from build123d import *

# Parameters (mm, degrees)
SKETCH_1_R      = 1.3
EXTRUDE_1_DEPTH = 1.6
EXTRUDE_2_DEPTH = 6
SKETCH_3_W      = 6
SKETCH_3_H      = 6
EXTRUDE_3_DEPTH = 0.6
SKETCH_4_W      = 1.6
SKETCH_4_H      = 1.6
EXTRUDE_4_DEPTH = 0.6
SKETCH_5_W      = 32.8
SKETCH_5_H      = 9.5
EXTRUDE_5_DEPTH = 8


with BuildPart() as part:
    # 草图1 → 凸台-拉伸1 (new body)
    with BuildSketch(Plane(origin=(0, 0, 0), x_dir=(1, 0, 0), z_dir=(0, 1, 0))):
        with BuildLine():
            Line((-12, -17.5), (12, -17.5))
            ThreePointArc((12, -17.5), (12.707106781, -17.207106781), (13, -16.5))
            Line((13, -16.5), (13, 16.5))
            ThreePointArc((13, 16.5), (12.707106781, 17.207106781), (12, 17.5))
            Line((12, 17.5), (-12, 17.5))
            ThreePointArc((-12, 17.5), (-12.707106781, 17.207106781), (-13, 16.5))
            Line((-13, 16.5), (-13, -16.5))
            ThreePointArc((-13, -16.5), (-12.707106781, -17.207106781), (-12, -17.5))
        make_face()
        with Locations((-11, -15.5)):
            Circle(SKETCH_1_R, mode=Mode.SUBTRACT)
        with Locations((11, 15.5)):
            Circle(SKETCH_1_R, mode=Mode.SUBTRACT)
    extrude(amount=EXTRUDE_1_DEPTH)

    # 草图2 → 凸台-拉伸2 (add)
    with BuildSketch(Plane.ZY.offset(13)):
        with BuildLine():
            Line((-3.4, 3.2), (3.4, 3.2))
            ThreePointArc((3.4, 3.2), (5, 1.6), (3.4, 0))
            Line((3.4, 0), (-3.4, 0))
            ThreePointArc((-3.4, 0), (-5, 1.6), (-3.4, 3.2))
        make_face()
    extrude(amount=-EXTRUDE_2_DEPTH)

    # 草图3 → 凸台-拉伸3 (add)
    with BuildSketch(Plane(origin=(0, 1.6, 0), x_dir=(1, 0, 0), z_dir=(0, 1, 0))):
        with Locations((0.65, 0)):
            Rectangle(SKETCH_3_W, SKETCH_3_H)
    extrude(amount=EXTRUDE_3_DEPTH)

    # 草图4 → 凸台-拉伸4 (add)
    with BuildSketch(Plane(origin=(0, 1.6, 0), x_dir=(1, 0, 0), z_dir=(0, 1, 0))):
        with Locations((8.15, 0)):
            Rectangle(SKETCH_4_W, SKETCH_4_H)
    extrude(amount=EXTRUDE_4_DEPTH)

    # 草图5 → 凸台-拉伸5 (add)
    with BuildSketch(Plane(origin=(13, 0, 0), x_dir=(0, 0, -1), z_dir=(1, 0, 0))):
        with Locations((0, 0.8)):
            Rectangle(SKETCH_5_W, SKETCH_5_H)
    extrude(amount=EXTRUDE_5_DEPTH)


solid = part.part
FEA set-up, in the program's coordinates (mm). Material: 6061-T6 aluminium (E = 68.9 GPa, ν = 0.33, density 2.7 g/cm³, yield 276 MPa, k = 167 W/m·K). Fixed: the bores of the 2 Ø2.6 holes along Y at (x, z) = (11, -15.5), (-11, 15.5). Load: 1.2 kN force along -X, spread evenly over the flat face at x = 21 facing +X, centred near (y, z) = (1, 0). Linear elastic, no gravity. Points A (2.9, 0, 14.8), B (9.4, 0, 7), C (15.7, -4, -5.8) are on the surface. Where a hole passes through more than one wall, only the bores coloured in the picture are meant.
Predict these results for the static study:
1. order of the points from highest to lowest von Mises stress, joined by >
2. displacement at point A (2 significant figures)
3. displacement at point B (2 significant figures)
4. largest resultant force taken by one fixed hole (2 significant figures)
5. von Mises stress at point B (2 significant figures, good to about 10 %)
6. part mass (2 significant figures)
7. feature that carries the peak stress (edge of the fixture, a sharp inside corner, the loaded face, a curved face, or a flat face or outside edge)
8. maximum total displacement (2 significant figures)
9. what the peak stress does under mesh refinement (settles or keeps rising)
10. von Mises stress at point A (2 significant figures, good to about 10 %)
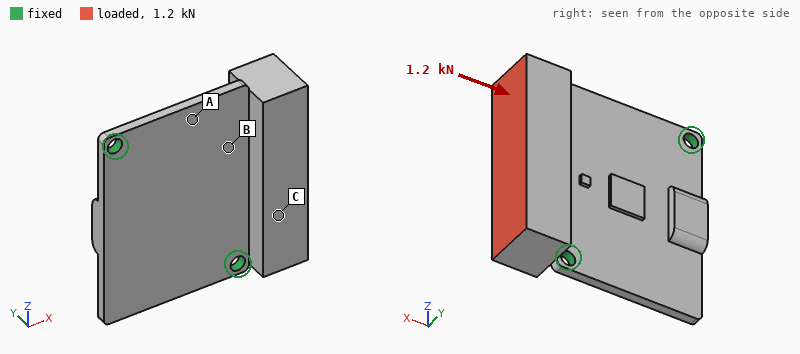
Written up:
A > B > C
9.9 µm
12 µm
600 N
23 MPa
11 g
edge of the fixture
17 µm
keeps rising
37 MPa
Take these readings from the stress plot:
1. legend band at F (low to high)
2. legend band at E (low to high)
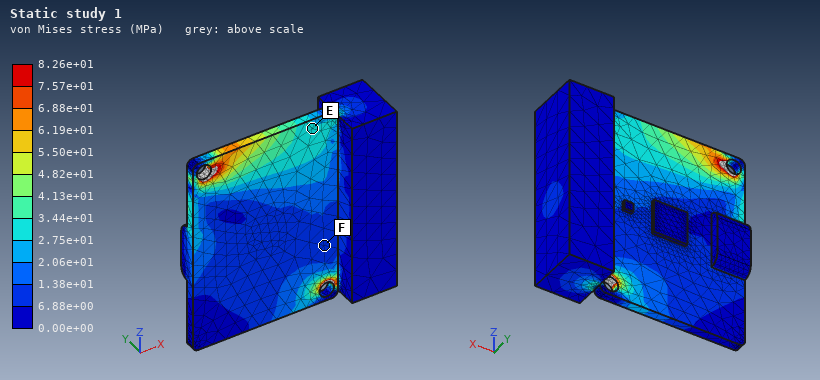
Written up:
6.88e+00 to 1.38e+01 MPa
2.75e+01 to 3.44e+01 MPa
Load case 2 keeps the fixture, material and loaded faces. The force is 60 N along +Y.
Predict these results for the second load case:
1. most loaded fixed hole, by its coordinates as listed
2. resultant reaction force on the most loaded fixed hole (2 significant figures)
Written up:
(11, -15.5)
52 N
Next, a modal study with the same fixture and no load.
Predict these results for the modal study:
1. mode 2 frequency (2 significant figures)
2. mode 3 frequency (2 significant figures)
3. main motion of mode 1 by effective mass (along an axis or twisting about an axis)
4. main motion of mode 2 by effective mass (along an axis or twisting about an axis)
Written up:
3500 Hz
5800 Hz
along Y
along Y
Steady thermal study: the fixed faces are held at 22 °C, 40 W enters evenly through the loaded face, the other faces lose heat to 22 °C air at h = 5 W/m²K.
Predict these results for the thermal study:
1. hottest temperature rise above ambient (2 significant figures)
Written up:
65 K
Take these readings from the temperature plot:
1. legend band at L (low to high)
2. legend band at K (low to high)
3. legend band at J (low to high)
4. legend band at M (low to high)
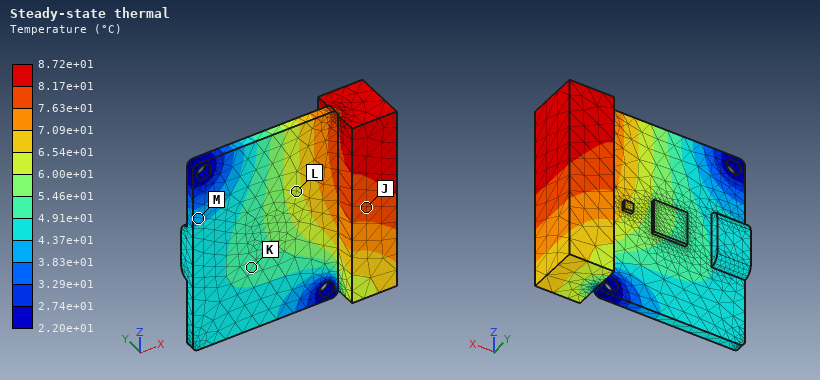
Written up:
6.00e+01 to 6.54e+01 °C
4.91e+01 to 5.46e+01 °C
7.63e+01 to 8.17e+01 °C
3.83e+01 to 4.37e+01 °C
